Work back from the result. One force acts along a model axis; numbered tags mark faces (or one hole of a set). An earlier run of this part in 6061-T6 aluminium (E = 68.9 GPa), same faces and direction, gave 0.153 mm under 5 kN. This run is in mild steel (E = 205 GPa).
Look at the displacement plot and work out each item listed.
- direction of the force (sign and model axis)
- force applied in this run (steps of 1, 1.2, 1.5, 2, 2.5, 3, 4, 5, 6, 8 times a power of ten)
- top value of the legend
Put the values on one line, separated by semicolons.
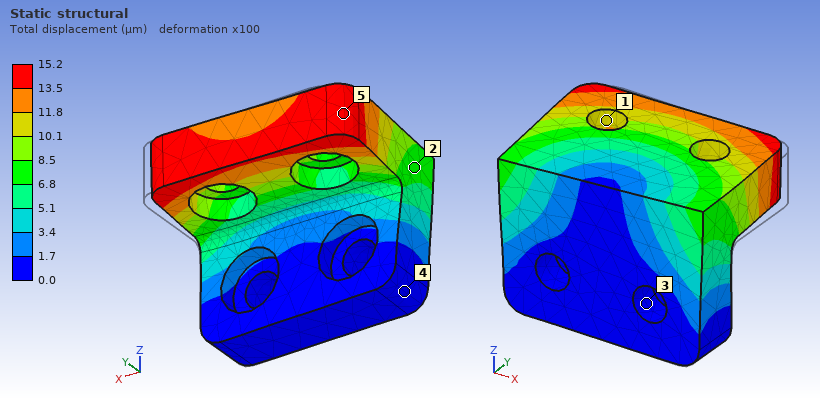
-X; 1.5 kN; 15.2 µm
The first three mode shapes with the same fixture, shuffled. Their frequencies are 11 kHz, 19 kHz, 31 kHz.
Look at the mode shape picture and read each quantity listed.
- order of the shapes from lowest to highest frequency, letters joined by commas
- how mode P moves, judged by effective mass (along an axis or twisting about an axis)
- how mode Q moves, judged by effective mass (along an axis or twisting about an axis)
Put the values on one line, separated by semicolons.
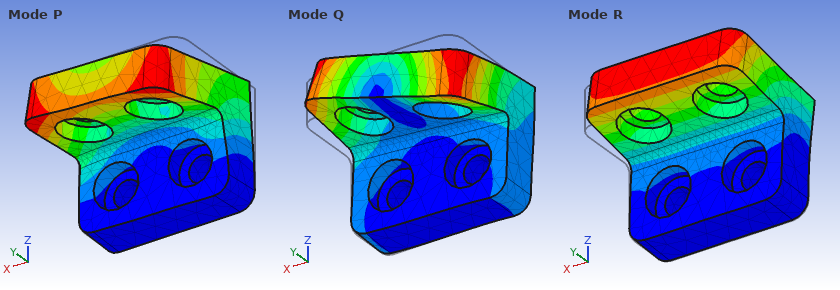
R, P, Q; along X; along X
